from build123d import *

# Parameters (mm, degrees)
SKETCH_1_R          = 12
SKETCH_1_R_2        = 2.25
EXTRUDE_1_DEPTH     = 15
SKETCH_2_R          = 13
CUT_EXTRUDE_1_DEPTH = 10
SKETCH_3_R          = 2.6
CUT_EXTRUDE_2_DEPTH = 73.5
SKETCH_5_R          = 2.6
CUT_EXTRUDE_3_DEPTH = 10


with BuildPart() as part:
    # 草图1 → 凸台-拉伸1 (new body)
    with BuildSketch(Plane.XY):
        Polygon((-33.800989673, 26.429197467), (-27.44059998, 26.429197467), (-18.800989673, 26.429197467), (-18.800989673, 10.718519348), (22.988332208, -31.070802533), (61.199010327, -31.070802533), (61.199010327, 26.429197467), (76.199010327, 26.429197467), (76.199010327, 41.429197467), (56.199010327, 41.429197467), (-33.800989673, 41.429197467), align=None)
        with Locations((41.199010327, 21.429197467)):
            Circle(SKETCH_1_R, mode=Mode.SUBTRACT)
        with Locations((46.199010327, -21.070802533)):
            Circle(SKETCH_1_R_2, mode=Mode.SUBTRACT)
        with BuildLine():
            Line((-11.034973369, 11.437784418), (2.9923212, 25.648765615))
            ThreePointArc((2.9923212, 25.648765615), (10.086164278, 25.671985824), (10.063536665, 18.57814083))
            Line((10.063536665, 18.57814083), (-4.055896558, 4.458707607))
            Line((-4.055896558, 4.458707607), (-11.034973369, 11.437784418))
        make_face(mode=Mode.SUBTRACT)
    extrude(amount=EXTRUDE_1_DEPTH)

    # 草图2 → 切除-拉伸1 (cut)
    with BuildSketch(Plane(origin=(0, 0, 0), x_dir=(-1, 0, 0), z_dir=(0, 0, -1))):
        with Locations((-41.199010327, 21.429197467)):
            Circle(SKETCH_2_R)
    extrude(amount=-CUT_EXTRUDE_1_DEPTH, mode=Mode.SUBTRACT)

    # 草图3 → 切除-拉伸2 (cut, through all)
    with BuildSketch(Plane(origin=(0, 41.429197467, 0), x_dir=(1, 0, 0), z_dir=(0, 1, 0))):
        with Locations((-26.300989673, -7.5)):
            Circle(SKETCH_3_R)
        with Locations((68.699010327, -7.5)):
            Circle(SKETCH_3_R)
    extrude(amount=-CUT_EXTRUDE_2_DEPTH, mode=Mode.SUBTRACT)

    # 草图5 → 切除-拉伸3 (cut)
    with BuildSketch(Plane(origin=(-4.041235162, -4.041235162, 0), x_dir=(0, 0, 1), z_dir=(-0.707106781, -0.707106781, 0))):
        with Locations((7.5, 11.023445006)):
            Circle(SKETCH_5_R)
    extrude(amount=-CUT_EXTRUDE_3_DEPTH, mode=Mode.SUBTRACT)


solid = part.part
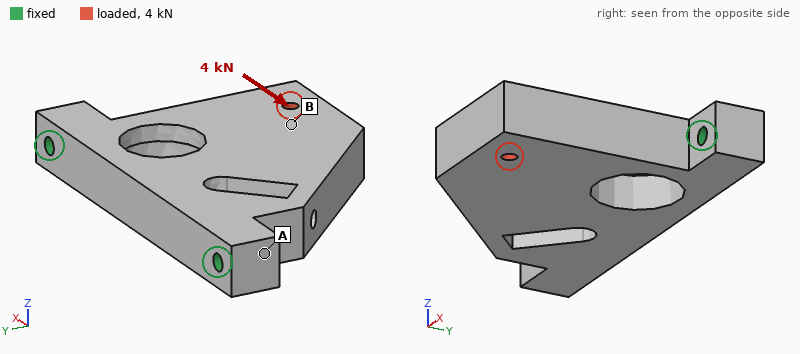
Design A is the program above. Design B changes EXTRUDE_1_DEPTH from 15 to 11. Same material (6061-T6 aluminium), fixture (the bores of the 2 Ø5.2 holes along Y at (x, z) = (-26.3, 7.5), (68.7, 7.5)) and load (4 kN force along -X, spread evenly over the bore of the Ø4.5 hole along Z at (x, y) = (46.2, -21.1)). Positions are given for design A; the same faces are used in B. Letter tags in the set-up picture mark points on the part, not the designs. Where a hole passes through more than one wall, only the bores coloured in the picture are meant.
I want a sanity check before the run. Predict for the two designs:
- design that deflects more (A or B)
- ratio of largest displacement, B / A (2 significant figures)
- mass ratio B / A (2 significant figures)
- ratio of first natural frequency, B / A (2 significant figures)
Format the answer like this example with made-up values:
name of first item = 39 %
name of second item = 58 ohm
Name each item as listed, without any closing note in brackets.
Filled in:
design that deflects more = B
ratio of largest displacement, B / A = 1.4
mass ratio B / A = 0.73
ratio of first natural frequency, B / A = 0.81
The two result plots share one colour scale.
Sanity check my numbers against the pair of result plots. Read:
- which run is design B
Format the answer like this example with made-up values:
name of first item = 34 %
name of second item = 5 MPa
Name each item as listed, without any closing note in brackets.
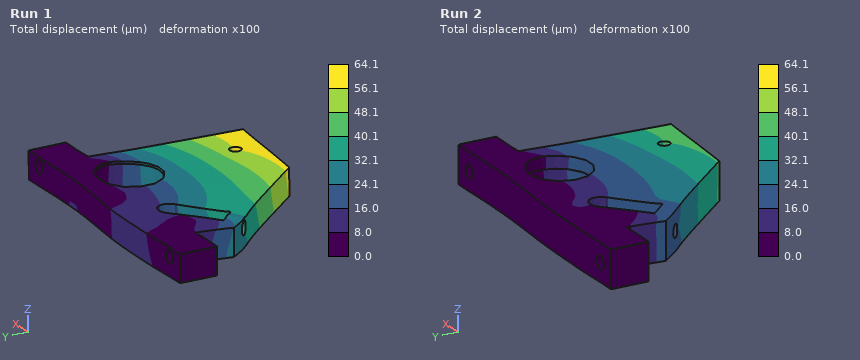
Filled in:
which run is design B = Run 1
